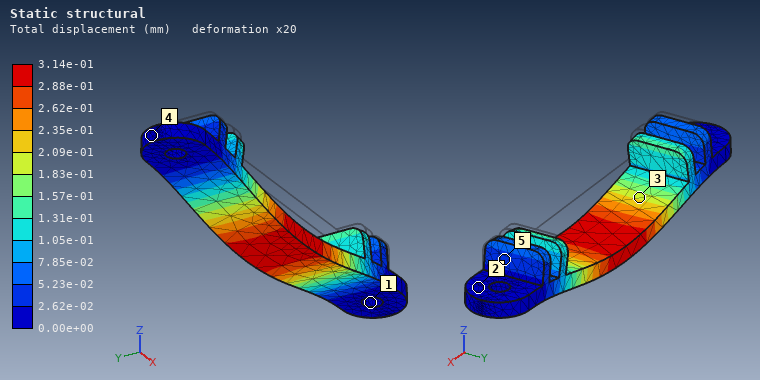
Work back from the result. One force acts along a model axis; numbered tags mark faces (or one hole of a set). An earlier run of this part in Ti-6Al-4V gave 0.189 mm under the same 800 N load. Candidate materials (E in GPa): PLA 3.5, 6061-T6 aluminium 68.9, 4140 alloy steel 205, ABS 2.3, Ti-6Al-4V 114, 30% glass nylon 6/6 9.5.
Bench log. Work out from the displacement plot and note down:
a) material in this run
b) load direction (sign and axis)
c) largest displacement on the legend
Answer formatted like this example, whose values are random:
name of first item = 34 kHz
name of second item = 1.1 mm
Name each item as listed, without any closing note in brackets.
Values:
material in this run = 6061-T6 aluminium
load direction = -Z
largest displacement on the legend = 3.14e-01 mm
